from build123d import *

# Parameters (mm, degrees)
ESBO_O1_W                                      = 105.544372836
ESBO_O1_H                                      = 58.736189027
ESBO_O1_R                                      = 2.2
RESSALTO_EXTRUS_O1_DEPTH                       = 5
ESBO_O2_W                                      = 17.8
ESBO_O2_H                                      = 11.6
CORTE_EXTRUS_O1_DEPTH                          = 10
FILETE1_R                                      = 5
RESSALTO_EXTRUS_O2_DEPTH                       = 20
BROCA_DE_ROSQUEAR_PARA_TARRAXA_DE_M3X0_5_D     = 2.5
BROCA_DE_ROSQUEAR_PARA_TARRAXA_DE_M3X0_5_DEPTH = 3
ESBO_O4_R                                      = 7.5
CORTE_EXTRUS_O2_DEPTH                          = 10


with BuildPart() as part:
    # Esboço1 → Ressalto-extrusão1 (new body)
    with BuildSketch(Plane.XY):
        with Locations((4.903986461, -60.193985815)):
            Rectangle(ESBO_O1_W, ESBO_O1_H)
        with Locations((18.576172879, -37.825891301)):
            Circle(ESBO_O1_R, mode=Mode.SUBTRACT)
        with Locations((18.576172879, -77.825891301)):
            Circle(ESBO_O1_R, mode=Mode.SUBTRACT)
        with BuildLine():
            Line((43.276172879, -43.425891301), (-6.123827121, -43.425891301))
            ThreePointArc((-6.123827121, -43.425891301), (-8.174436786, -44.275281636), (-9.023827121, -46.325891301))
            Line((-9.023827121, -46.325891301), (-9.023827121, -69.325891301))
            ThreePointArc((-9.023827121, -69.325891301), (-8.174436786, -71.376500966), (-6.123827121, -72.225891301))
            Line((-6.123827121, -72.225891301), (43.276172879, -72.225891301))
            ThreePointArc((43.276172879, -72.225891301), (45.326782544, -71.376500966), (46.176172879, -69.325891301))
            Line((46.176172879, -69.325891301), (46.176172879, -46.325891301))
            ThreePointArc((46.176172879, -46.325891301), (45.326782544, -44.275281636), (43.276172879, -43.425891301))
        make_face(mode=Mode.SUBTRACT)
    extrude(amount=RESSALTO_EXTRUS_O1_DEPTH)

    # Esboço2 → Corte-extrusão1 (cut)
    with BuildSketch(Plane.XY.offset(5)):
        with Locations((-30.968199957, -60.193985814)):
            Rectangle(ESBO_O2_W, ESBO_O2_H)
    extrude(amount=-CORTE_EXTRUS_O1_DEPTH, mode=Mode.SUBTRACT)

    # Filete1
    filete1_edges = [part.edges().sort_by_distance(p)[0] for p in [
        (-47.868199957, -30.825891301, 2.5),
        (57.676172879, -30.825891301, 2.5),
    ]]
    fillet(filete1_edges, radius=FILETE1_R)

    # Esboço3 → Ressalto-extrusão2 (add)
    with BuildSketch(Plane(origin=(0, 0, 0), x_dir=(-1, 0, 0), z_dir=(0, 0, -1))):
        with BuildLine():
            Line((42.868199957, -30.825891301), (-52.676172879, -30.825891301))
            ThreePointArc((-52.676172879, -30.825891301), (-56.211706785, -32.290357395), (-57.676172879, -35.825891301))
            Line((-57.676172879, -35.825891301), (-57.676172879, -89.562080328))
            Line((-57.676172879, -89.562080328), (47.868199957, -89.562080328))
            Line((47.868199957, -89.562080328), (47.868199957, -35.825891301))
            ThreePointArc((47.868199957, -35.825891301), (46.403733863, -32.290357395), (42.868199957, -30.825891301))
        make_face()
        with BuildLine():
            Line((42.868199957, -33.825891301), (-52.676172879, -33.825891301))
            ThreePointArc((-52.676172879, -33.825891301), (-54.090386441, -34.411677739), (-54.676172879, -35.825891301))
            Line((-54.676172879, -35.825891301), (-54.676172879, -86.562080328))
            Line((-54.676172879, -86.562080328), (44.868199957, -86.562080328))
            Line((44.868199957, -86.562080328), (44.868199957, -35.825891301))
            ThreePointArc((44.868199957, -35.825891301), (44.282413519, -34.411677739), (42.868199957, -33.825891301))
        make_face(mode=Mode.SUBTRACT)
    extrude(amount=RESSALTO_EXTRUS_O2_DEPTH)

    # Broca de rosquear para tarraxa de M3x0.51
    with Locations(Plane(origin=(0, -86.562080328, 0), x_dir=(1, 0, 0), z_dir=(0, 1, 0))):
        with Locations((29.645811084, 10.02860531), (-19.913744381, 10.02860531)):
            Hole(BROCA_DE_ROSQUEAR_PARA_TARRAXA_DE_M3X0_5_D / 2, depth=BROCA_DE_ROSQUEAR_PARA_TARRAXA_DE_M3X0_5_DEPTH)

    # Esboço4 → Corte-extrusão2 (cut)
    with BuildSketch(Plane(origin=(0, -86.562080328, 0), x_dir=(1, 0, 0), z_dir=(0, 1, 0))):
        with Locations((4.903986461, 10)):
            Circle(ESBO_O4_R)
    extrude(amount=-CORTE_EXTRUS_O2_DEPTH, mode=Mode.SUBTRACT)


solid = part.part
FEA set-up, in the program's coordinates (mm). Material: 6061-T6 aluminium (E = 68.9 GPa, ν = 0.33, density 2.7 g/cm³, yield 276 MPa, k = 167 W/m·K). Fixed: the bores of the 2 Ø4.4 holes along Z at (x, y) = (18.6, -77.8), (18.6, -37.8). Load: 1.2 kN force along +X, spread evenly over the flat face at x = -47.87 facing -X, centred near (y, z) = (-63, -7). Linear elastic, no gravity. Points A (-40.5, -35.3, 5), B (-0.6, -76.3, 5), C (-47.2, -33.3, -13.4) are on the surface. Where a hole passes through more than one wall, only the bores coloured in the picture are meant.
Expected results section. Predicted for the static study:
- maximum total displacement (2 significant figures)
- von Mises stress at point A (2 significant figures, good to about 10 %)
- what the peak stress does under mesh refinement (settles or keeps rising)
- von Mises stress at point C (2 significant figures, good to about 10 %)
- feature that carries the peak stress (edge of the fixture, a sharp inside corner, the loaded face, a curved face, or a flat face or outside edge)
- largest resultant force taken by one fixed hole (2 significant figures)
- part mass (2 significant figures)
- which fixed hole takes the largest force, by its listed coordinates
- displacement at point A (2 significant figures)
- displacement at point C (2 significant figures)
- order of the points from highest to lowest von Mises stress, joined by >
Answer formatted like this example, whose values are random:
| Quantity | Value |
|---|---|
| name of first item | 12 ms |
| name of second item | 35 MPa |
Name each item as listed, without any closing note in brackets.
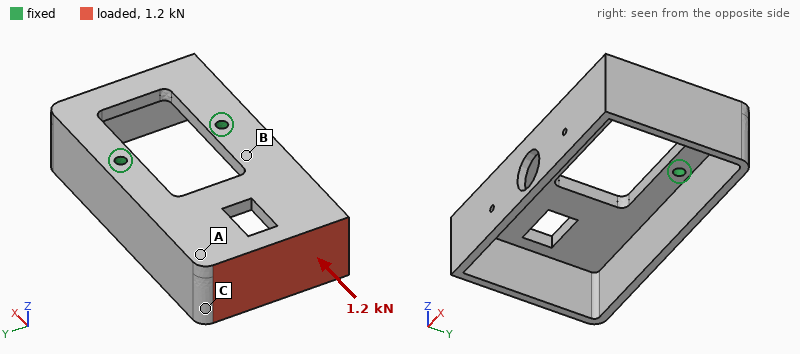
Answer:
| Quantity | Value |
|---|---|
| maximum total displacement | 0.22 mm |
| von Mises stress at point A | 11 MPa |
| what the peak stress does under mesh refinement | keeps rising |
| von Mises stress at point C | 34 MPa |
| feature that carries the peak stress | edge of the fixture |
| largest resultant force taken by one fixed hole | 720 N |
| part mass | 110 g |
| which fixed hole takes the largest force, by its listed coordinates | (18.6, -77.8) |
| displacement at point A | 0.11 mm |
| displacement at point C | 0.12 mm |
| order of the points from highest to lowest von Mises stress, joined by > | C > A > B |
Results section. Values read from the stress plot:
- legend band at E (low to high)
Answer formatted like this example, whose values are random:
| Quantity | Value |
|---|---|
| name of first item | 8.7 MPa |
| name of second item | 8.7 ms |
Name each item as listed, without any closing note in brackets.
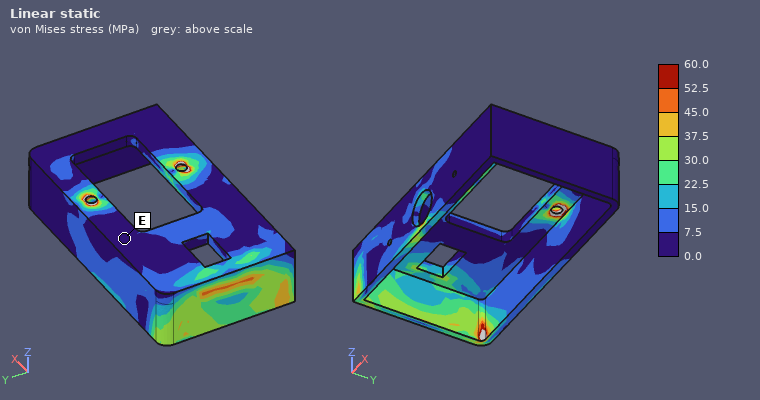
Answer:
| Quantity | Value |
|---|---|
| legend band at E | 0.0 to 7.5 MPa |
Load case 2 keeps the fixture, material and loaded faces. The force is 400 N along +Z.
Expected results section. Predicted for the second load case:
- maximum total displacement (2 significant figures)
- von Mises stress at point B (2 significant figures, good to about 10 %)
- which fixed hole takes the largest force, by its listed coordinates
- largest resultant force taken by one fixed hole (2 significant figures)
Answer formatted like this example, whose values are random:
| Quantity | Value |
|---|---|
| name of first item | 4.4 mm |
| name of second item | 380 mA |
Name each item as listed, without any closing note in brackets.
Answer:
| Quantity | Value |
|---|---|
| maximum total displacement | 0.38 mm |
| von Mises stress at point B | 20 MPa |
| which fixed hole takes the largest force, by its listed coordinates | (18.6, -77.8) |
| largest resultant force taken by one fixed hole | 220 N |
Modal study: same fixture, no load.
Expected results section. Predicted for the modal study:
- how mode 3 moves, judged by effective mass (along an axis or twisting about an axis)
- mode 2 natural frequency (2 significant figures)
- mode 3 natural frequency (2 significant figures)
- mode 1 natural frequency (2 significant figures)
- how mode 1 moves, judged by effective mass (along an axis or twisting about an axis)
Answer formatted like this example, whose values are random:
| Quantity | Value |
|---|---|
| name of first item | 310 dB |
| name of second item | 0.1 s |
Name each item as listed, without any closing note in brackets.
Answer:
| Quantity | Value |
|---|---|
| how mode 3 moves, judged by effective mass | along Y |
| mode 2 natural frequency | 1600 Hz |
| mode 3 natural frequency | 2900 Hz |
| mode 1 natural frequency | 960 Hz |
| how mode 1 moves, judged by effective mass | along Z |
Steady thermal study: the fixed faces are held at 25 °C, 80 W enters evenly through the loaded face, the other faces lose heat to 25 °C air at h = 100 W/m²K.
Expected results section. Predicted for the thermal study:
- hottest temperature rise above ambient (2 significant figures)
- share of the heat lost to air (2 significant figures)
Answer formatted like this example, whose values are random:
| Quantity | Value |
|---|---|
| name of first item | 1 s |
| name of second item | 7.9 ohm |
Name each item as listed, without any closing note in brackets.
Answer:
| Quantity | Value |
|---|---|
| hottest temperature rise above ambient | 78 K |
| share of the heat lost to air | 63 % |
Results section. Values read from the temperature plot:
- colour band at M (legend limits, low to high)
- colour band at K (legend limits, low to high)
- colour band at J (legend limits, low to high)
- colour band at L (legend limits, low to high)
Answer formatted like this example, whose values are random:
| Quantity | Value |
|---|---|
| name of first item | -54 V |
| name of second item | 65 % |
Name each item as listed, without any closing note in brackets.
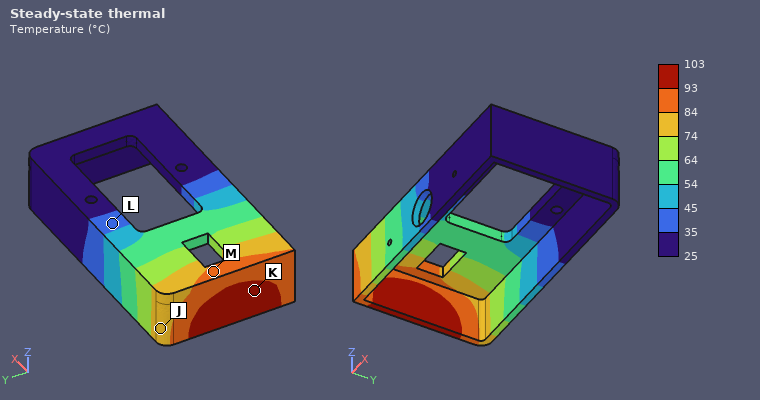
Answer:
| Quantity | Value |
|---|---|
| colour band at M | 84 to 93 °C |
| colour band at K | 93 to 103 °C |
| colour band at J | 74 to 84 °C |
| colour band at L | 35 to 45 °C |
